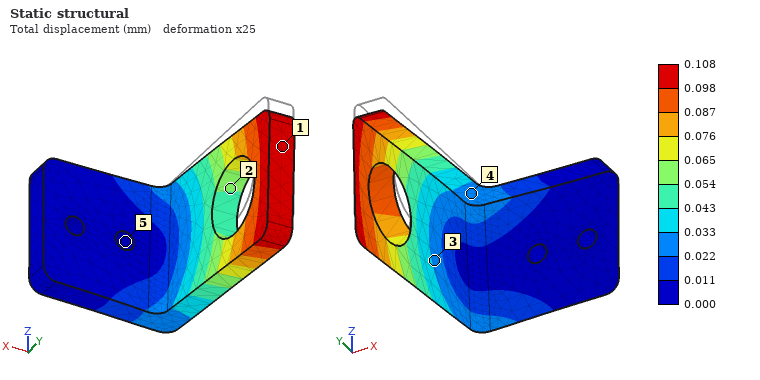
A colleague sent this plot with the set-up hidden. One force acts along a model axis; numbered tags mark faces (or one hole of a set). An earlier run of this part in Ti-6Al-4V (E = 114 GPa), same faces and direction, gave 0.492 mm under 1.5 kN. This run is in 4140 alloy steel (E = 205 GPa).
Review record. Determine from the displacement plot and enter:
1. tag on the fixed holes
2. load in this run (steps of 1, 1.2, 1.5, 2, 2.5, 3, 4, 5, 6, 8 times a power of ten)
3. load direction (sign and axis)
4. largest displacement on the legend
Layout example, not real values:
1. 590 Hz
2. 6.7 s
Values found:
1. 5
2. 600 N
3. -Z
4. 0.108 mm
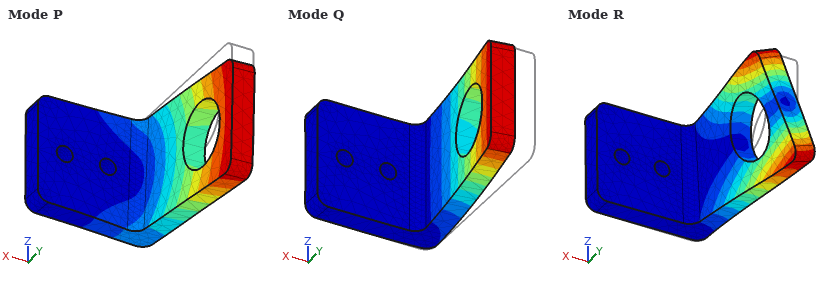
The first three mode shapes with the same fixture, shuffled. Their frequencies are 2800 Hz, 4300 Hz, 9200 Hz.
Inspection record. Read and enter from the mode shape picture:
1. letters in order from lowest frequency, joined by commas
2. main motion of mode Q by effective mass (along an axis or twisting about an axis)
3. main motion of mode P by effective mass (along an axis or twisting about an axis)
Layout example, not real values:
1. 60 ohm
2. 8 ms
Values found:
1. Q, P, R
2. along X
3. along Z
